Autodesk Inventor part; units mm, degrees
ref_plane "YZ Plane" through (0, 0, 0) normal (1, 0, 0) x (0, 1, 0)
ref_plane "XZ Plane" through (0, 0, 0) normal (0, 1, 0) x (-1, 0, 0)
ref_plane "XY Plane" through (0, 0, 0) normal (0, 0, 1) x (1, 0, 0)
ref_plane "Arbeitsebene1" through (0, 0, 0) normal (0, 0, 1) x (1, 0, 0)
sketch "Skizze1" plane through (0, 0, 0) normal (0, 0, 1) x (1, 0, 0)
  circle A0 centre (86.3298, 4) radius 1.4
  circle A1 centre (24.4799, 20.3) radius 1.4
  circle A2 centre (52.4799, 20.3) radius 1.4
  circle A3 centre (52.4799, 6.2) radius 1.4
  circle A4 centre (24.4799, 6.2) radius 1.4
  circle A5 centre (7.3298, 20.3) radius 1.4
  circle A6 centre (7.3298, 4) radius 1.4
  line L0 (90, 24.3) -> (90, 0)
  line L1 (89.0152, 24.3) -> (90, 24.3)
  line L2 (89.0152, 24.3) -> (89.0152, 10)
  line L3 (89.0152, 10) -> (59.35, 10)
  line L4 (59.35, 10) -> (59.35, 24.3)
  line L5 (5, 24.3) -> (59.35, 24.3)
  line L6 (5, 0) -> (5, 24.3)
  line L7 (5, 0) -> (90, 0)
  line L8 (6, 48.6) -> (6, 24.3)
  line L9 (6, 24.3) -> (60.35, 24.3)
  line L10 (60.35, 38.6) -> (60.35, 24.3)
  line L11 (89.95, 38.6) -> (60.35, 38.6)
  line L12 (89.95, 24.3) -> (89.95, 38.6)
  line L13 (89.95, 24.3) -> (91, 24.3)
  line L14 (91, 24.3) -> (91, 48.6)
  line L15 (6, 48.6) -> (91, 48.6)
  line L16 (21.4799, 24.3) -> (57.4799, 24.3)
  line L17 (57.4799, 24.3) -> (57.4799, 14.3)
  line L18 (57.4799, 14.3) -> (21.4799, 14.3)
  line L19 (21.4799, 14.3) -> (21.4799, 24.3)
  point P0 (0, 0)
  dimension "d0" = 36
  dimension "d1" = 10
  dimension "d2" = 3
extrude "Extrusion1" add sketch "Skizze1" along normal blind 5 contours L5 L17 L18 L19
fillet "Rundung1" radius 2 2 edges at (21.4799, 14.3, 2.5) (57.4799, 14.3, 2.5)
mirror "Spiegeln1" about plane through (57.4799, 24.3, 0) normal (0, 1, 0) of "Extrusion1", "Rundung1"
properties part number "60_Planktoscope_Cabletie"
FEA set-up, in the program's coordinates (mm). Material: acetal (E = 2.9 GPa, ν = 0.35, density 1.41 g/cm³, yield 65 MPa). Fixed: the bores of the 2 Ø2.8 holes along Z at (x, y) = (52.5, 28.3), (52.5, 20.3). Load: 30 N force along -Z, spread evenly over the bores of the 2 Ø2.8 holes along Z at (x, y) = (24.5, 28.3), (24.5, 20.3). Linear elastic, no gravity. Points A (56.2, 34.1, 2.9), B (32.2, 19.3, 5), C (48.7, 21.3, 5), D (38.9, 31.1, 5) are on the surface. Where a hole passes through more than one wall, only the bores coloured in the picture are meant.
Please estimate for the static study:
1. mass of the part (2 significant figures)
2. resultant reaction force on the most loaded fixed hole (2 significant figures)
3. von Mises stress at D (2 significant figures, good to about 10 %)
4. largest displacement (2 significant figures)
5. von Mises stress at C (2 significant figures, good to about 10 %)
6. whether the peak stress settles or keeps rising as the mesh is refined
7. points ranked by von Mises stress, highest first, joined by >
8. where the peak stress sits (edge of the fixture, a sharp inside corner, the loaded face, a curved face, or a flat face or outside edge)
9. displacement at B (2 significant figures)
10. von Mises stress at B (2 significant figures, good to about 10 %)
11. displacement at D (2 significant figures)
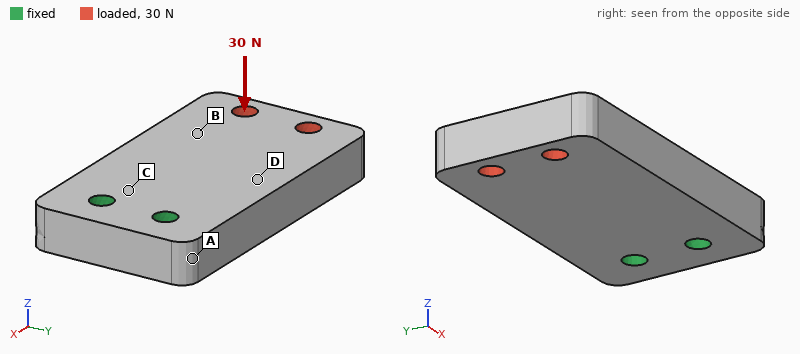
4.9 g
15 N
5.1 MPa
0.42 mm
9.3 MPa
keeps rising
C > D > B > A
edge of the fixture
0.22 mm
2.8 MPa
0.11 mm
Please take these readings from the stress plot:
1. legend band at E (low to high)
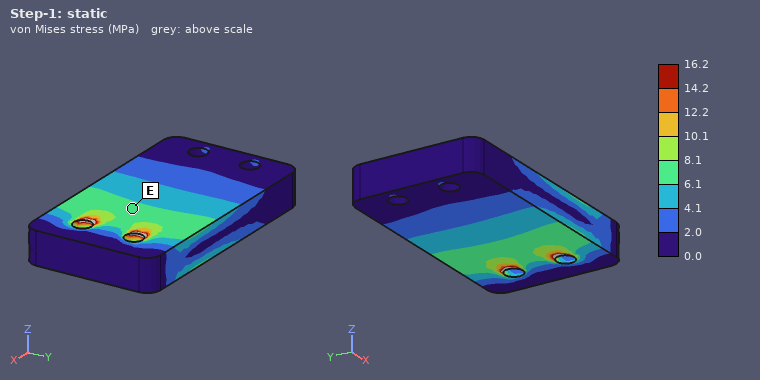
6.1 to 8.1 MPa
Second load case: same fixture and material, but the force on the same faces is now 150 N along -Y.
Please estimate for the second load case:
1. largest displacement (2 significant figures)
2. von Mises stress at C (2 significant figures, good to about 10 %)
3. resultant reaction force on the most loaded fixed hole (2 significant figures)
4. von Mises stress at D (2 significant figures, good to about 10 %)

0.26 mm
9.5 MPa
410 N
4.9 MPa
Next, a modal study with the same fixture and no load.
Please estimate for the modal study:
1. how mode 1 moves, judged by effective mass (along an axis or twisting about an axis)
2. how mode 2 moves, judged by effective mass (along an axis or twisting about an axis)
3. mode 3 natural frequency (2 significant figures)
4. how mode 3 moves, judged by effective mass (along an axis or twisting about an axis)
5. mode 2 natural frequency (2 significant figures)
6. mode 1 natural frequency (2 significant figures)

along Z
along Y
3600 Hz
twisting about X
3200 Hz
1200 Hz
